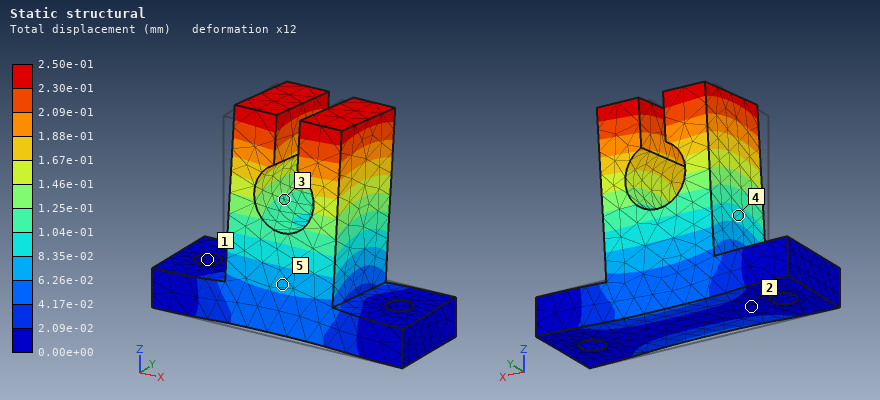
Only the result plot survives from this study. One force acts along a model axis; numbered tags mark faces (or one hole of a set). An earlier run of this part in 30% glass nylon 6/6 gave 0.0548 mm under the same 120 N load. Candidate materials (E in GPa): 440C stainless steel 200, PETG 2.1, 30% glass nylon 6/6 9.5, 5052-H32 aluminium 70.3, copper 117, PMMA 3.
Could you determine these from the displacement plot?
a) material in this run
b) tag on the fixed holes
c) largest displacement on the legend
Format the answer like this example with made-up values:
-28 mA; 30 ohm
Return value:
PETG; 1; 2.50e-01 mm
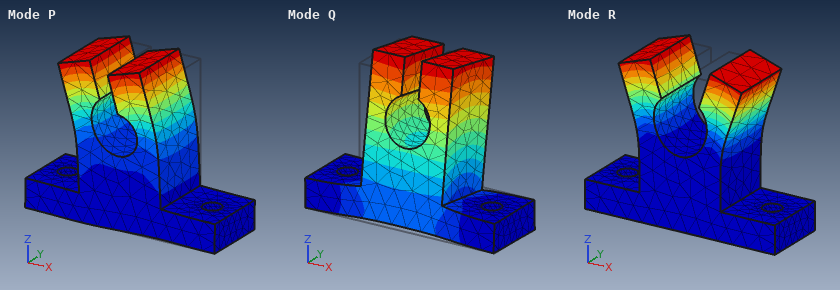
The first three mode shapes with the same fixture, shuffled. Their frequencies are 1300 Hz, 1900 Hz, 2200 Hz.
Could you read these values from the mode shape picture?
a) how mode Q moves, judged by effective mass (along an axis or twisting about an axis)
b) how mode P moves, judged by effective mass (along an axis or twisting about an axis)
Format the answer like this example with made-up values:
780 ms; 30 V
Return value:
along Y; along X
